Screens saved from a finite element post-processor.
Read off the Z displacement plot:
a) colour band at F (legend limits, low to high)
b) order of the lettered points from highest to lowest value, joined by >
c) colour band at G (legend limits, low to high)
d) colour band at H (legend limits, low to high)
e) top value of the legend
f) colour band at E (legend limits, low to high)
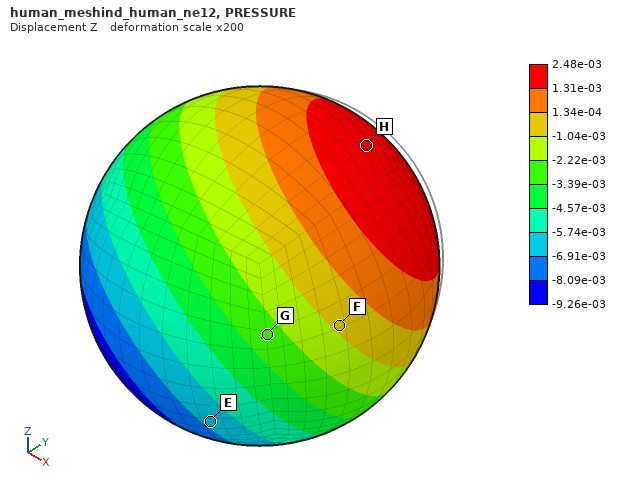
-1.04e-03 to 1.34e-04
H > F > G > E
-3.39e-03 to -2.22e-03
1.31e-03 to 2.48e-03
2.48e-03
-6.91e-03 to -5.74e-03
